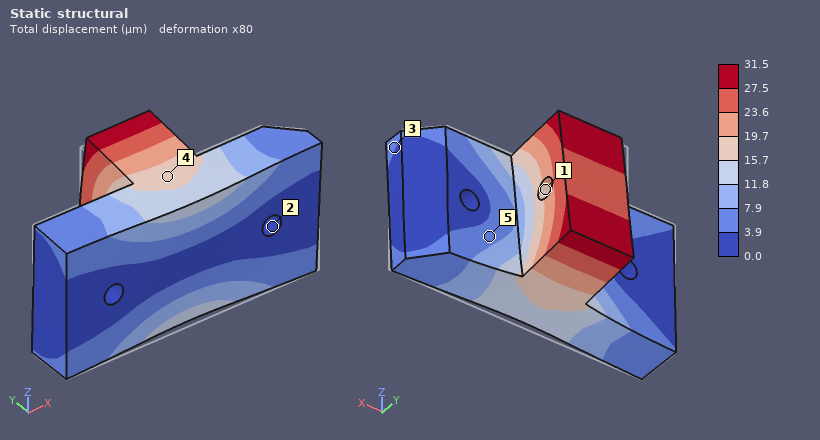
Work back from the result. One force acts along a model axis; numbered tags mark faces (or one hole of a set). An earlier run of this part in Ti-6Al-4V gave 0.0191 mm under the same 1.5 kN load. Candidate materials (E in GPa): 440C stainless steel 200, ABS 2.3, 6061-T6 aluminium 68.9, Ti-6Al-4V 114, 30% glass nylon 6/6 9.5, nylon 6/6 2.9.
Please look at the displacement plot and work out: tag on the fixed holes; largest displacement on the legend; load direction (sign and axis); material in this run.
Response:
2
31.5 µm
+Z
6061-T6 aluminium
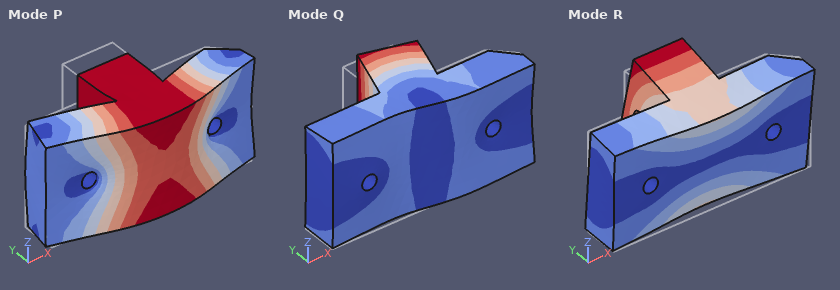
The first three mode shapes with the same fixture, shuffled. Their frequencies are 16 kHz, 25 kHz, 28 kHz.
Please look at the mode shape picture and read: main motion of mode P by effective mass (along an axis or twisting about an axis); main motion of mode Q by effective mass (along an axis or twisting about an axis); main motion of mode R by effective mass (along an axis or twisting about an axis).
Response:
along Y
along X
along Z
